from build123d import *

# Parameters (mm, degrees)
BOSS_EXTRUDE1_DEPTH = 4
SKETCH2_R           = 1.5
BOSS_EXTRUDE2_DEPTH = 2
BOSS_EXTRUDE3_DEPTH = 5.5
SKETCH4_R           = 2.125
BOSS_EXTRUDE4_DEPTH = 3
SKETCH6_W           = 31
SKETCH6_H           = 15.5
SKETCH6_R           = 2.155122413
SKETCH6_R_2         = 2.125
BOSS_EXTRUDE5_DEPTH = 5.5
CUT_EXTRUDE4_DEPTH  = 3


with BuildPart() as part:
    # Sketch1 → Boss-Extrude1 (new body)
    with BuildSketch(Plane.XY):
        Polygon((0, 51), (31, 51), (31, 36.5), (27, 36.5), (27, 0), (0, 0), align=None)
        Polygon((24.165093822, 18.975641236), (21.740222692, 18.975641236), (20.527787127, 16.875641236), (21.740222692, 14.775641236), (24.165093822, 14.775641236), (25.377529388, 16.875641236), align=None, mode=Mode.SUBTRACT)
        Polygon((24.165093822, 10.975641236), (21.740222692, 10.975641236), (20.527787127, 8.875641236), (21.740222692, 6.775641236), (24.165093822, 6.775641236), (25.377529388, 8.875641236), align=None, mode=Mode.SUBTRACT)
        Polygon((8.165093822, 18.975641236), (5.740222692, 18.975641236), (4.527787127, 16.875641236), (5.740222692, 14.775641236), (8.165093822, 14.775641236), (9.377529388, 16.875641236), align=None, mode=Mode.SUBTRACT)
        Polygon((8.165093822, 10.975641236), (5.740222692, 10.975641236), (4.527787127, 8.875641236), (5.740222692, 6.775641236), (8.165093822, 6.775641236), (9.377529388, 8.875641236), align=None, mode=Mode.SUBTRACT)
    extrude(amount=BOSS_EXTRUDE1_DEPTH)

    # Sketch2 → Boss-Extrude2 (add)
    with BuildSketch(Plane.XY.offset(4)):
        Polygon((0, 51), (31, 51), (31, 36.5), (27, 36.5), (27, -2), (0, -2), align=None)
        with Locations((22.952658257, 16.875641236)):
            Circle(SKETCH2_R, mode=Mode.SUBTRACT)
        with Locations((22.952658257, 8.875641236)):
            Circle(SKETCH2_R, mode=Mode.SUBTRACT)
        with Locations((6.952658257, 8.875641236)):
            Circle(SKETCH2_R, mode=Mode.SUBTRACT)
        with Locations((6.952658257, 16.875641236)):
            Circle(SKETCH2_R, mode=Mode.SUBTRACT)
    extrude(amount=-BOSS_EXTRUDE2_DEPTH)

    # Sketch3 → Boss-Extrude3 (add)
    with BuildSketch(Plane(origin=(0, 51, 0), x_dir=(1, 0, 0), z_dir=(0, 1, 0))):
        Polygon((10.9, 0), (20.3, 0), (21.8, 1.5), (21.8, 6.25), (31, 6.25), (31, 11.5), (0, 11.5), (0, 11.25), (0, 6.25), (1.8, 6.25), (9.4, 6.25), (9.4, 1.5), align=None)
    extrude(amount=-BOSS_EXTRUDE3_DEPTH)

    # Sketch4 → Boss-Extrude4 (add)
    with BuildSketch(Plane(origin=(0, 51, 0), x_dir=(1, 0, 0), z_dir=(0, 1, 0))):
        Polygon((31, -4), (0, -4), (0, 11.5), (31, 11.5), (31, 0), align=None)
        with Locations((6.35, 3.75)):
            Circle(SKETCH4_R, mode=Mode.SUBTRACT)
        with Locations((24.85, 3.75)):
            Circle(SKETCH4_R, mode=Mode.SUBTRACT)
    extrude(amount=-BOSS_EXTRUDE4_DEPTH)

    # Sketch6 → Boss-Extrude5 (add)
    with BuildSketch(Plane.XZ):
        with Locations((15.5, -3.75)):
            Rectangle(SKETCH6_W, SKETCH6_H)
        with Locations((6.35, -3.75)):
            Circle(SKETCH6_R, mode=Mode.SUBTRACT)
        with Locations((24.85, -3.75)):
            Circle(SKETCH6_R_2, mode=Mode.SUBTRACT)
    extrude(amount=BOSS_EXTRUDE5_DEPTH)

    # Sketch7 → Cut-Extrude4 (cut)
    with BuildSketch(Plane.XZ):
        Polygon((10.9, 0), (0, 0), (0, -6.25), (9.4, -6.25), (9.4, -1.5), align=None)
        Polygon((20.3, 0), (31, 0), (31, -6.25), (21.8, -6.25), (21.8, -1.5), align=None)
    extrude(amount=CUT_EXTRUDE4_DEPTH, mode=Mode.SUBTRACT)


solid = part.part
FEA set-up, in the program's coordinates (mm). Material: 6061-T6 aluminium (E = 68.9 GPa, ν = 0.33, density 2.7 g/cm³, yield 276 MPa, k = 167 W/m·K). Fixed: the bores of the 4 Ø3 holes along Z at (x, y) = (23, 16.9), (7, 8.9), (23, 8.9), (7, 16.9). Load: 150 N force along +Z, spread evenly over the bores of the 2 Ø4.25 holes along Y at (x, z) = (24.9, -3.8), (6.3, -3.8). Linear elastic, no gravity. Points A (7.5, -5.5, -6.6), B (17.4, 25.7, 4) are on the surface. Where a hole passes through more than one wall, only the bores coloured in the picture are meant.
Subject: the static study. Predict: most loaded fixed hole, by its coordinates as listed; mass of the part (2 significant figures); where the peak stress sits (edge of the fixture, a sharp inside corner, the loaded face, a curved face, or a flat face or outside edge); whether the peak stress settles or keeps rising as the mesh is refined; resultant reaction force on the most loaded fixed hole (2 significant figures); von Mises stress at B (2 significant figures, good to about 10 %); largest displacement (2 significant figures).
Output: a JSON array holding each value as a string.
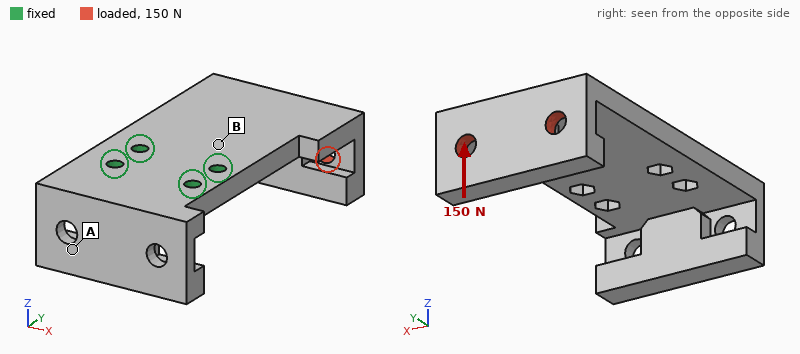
["(7, 16.9)", "25 g", "edge of the fixture", "keeps rising", "370 N", "46 MPa", "0.26 mm"]
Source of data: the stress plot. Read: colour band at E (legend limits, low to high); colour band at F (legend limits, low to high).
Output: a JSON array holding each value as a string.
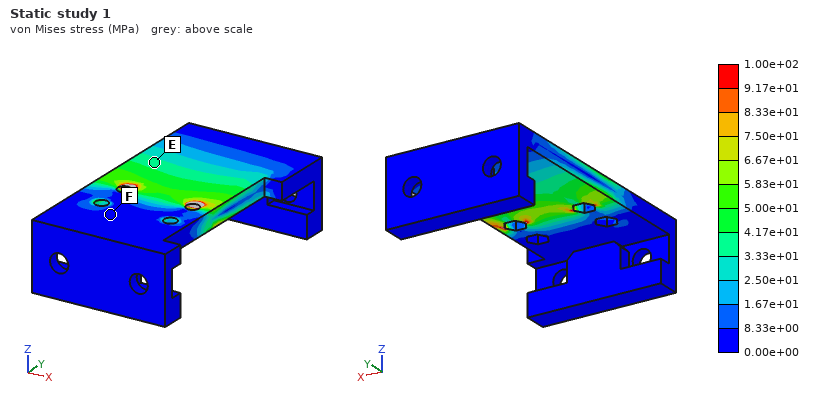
["3.33e+01 to 4.17e+01 MPa", "0.00e+00 to 8.33e+00 MPa"]
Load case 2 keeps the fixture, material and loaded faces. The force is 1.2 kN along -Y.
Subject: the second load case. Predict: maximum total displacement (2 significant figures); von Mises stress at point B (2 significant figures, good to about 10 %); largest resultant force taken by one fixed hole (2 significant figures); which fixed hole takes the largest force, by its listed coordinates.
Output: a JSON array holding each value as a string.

["0.57 mm", "77 MPa", "630 N", "(7, 8.9)"]
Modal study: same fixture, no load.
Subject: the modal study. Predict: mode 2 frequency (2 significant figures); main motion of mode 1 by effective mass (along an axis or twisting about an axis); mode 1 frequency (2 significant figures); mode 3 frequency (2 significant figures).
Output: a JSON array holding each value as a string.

["3800 Hz", "along Z", "1500 Hz", "4900 Hz"]
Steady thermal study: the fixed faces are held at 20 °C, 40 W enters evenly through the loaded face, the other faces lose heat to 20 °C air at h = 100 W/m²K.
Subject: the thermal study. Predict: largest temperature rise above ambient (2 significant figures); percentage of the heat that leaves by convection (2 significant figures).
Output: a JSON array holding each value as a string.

["67 K", "33 %"]
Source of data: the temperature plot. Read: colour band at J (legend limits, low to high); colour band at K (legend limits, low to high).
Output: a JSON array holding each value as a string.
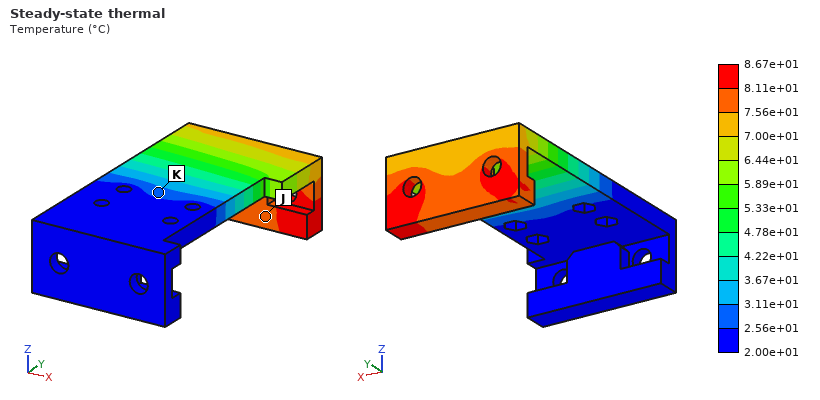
["7.56e+01 to 8.11e+01 °C", "2.56e+01 to 3.11e+01 °C"]
